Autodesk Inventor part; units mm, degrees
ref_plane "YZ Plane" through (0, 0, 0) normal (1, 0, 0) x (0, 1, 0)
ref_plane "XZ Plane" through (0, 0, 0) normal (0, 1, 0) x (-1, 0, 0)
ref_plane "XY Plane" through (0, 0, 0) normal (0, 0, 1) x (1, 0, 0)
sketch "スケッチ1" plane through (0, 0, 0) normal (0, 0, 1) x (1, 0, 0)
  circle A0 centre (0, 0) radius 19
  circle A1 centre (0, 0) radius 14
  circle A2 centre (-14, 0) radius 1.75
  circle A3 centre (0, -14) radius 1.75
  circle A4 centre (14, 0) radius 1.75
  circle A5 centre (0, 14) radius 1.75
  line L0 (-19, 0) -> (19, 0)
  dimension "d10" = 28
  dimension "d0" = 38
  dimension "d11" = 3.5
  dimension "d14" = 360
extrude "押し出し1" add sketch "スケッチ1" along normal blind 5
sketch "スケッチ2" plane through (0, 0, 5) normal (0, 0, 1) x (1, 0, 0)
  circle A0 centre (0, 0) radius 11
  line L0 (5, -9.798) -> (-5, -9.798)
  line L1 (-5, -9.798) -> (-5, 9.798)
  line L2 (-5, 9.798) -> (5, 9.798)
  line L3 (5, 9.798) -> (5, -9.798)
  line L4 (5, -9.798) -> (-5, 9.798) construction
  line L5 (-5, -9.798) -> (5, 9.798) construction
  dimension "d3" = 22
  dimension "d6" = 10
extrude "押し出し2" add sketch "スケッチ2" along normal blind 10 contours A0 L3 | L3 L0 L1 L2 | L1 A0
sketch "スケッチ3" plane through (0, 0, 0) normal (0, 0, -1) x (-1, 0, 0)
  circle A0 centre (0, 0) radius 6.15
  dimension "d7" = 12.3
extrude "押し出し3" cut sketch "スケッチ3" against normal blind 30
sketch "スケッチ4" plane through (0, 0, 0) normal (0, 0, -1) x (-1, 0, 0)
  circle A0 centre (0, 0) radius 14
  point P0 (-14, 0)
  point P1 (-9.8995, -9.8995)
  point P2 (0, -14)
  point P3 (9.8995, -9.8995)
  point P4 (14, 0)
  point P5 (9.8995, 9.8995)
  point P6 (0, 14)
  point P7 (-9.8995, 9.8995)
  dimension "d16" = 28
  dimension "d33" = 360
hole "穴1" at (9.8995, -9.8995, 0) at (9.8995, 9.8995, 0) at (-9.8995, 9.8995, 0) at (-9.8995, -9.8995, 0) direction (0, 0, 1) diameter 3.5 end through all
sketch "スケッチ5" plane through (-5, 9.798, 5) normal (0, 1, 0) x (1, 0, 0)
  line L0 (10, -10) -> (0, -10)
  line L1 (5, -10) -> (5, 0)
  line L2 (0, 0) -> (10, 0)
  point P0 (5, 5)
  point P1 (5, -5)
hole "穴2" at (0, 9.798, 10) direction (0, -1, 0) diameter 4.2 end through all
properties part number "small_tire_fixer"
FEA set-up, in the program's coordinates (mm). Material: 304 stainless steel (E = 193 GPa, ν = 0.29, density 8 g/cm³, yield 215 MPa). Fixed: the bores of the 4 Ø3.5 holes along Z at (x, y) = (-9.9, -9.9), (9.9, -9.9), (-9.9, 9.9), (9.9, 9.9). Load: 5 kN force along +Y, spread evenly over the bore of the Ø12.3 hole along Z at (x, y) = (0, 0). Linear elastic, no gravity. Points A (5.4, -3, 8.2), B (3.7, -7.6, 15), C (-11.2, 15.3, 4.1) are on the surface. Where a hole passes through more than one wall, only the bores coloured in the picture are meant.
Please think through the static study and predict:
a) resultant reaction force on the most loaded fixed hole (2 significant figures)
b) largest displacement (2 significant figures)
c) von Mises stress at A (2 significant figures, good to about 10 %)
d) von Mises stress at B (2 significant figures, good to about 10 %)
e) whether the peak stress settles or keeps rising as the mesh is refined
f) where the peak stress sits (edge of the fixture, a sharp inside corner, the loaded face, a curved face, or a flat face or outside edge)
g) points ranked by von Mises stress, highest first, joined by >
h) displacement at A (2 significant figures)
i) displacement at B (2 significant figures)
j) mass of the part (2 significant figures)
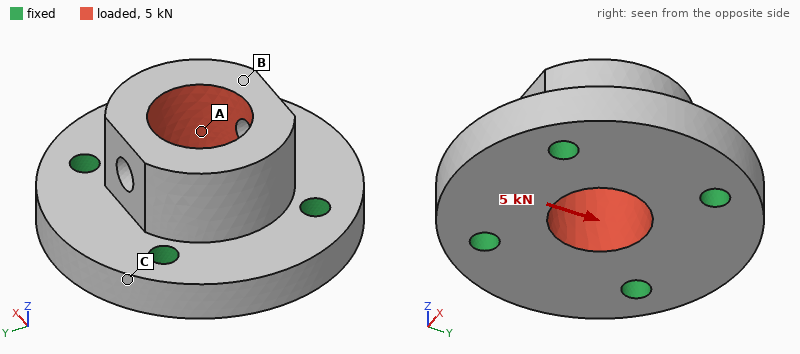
1.4 kN
4.8 µm
34 MPa
22 MPa
keeps rising
a sharp inside corner
A > B > C
2.2 µm
4.3 µm
58 g
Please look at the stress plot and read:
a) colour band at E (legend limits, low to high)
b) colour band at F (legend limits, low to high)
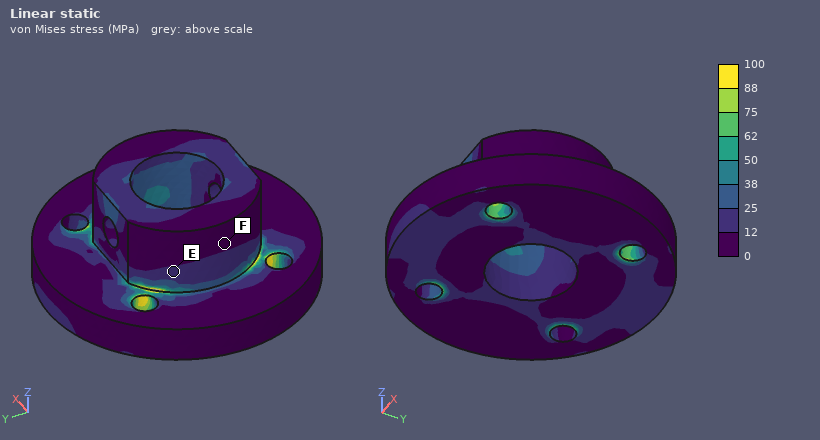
12 to 25 MPa
0 to 12 MPa
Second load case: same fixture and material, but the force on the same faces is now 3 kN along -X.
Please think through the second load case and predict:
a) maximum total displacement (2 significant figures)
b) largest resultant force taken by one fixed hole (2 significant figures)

3.2 µm
840 N
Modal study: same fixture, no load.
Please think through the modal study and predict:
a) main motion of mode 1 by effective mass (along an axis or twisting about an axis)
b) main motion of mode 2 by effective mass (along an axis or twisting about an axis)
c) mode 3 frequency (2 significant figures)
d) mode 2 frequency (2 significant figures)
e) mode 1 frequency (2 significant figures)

along X
along Y
37 kHz
34 kHz
32 kHz
